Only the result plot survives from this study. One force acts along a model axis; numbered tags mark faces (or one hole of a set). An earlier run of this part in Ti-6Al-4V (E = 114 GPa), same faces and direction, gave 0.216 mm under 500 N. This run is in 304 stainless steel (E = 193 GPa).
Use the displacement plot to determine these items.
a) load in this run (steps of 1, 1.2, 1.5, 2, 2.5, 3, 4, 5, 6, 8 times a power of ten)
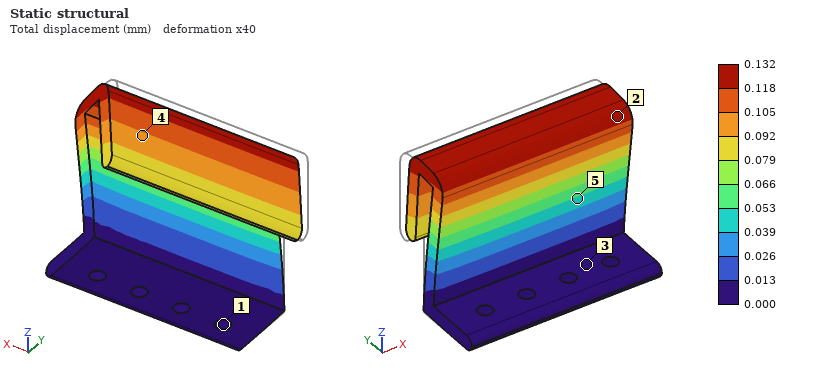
500 N
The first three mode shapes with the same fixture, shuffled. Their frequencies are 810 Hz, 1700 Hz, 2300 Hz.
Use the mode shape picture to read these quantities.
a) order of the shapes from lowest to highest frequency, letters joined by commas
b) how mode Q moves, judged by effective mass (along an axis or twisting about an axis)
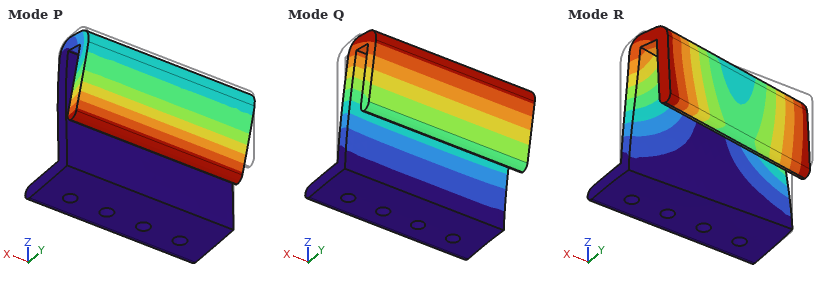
Q, R, P
along Y
